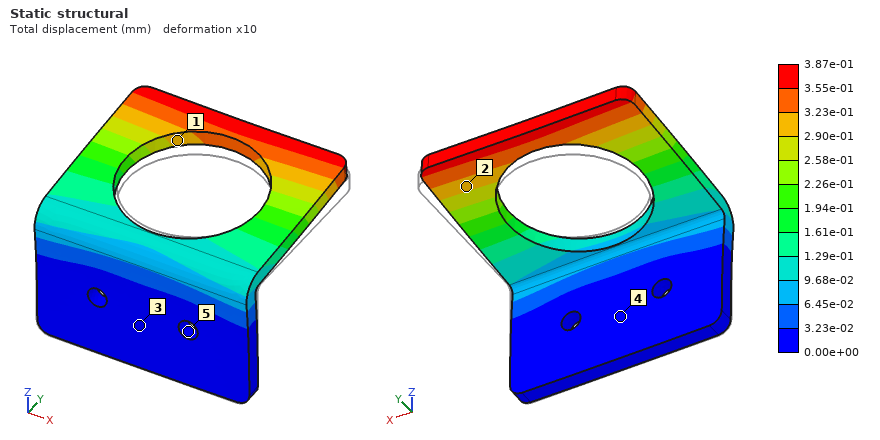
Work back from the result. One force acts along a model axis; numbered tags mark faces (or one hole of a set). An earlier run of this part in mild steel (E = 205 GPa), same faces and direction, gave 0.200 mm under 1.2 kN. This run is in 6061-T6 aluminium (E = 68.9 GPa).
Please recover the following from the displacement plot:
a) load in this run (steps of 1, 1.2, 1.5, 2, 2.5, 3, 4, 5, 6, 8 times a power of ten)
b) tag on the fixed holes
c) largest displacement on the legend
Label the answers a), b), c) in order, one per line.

a) 800 N
b) 5
c) 3.87e-01 mm
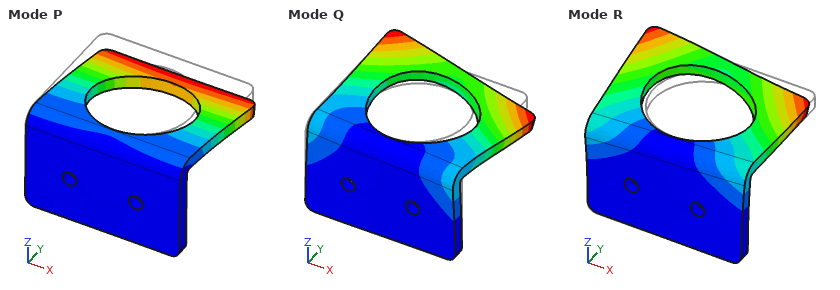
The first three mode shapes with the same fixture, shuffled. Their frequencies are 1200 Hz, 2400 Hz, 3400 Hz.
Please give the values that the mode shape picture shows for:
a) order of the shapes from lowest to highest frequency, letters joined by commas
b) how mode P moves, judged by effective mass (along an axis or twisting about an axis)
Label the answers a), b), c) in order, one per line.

a) P, R, Q
b) along Z
